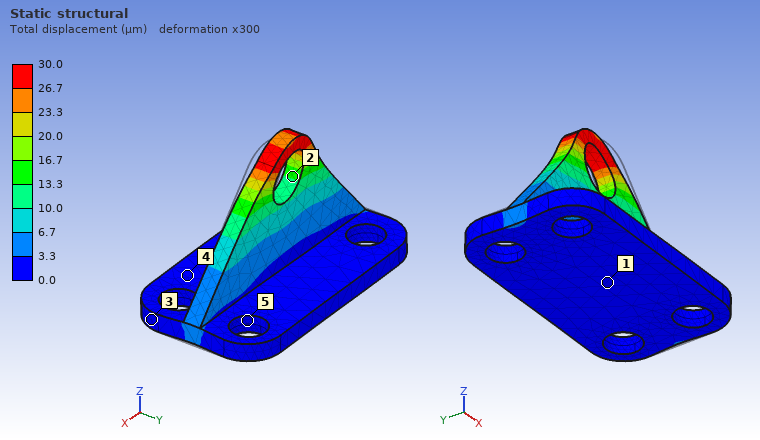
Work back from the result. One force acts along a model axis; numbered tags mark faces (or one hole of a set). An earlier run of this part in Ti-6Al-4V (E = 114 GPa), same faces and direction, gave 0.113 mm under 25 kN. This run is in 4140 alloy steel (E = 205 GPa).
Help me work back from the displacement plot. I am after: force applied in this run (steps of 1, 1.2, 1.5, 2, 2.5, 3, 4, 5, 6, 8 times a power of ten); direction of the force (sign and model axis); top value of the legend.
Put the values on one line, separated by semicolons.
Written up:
12 kN; -X; 30.0 µm
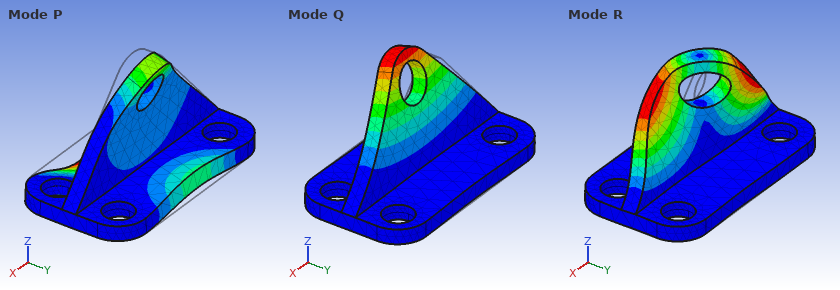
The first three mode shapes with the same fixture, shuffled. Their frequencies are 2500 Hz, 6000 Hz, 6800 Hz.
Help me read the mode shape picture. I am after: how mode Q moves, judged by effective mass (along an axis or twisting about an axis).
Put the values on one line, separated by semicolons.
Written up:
along Y
